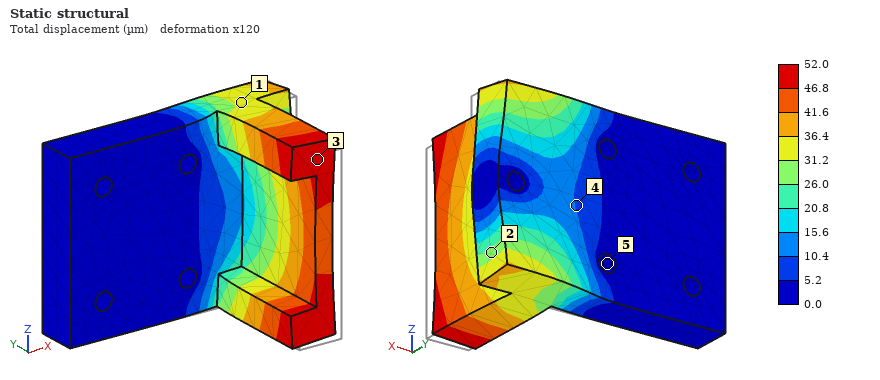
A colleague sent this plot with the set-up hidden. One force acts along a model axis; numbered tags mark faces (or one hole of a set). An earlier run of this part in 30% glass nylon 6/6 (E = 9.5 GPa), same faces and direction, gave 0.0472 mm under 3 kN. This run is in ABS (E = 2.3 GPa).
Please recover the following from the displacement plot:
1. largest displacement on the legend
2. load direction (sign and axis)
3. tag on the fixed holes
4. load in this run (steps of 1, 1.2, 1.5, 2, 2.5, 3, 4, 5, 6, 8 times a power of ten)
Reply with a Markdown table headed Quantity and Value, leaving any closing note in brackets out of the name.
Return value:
| Quantity | Value |
|---|---|
| largest displacement on the legend | 52.0 µm |
| load direction | +Y |
| tag on the fixed holes | 5 |
| load in this run | 800 N |
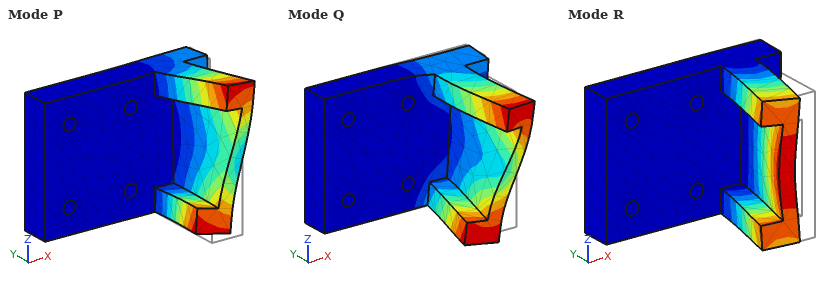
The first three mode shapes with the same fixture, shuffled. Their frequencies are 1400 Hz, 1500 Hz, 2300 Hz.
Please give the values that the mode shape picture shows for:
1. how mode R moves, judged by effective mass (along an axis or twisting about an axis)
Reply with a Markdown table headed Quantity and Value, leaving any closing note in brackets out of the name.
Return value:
| Quantity | Value |
|---|---|
| how mode R moves, judged by effective mass | along X |
